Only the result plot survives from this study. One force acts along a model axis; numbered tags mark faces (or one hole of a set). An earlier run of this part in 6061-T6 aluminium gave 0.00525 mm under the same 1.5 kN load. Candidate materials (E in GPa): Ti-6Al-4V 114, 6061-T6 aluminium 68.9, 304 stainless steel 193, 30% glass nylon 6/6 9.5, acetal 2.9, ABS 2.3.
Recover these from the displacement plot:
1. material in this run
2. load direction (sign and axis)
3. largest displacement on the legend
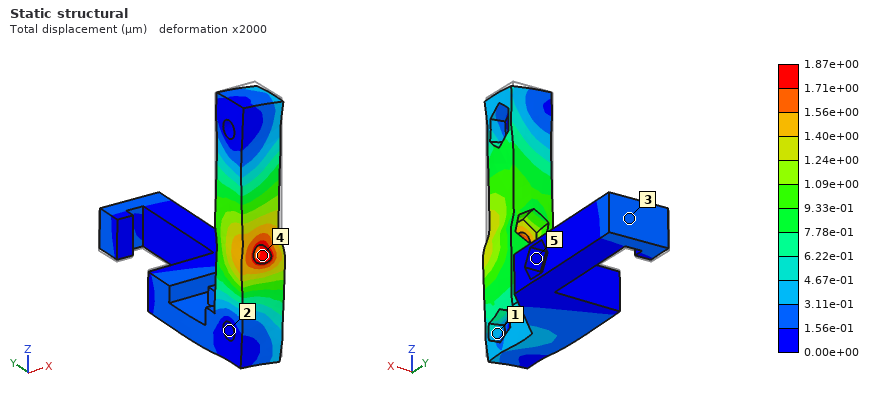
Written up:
304 stainless steel
-Z
1.87e+00 µm
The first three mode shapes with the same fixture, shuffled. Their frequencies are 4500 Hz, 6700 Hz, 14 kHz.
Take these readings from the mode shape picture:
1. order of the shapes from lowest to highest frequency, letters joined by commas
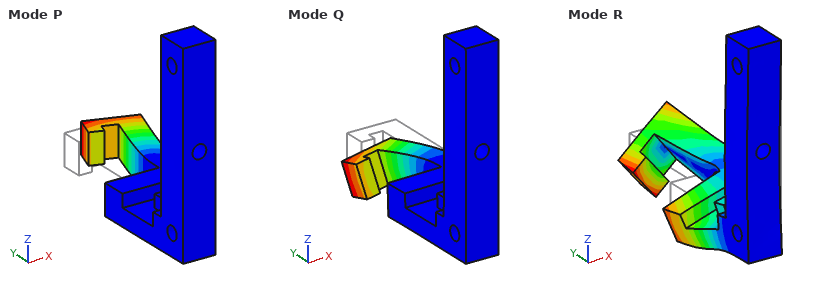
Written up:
P, Q, R
